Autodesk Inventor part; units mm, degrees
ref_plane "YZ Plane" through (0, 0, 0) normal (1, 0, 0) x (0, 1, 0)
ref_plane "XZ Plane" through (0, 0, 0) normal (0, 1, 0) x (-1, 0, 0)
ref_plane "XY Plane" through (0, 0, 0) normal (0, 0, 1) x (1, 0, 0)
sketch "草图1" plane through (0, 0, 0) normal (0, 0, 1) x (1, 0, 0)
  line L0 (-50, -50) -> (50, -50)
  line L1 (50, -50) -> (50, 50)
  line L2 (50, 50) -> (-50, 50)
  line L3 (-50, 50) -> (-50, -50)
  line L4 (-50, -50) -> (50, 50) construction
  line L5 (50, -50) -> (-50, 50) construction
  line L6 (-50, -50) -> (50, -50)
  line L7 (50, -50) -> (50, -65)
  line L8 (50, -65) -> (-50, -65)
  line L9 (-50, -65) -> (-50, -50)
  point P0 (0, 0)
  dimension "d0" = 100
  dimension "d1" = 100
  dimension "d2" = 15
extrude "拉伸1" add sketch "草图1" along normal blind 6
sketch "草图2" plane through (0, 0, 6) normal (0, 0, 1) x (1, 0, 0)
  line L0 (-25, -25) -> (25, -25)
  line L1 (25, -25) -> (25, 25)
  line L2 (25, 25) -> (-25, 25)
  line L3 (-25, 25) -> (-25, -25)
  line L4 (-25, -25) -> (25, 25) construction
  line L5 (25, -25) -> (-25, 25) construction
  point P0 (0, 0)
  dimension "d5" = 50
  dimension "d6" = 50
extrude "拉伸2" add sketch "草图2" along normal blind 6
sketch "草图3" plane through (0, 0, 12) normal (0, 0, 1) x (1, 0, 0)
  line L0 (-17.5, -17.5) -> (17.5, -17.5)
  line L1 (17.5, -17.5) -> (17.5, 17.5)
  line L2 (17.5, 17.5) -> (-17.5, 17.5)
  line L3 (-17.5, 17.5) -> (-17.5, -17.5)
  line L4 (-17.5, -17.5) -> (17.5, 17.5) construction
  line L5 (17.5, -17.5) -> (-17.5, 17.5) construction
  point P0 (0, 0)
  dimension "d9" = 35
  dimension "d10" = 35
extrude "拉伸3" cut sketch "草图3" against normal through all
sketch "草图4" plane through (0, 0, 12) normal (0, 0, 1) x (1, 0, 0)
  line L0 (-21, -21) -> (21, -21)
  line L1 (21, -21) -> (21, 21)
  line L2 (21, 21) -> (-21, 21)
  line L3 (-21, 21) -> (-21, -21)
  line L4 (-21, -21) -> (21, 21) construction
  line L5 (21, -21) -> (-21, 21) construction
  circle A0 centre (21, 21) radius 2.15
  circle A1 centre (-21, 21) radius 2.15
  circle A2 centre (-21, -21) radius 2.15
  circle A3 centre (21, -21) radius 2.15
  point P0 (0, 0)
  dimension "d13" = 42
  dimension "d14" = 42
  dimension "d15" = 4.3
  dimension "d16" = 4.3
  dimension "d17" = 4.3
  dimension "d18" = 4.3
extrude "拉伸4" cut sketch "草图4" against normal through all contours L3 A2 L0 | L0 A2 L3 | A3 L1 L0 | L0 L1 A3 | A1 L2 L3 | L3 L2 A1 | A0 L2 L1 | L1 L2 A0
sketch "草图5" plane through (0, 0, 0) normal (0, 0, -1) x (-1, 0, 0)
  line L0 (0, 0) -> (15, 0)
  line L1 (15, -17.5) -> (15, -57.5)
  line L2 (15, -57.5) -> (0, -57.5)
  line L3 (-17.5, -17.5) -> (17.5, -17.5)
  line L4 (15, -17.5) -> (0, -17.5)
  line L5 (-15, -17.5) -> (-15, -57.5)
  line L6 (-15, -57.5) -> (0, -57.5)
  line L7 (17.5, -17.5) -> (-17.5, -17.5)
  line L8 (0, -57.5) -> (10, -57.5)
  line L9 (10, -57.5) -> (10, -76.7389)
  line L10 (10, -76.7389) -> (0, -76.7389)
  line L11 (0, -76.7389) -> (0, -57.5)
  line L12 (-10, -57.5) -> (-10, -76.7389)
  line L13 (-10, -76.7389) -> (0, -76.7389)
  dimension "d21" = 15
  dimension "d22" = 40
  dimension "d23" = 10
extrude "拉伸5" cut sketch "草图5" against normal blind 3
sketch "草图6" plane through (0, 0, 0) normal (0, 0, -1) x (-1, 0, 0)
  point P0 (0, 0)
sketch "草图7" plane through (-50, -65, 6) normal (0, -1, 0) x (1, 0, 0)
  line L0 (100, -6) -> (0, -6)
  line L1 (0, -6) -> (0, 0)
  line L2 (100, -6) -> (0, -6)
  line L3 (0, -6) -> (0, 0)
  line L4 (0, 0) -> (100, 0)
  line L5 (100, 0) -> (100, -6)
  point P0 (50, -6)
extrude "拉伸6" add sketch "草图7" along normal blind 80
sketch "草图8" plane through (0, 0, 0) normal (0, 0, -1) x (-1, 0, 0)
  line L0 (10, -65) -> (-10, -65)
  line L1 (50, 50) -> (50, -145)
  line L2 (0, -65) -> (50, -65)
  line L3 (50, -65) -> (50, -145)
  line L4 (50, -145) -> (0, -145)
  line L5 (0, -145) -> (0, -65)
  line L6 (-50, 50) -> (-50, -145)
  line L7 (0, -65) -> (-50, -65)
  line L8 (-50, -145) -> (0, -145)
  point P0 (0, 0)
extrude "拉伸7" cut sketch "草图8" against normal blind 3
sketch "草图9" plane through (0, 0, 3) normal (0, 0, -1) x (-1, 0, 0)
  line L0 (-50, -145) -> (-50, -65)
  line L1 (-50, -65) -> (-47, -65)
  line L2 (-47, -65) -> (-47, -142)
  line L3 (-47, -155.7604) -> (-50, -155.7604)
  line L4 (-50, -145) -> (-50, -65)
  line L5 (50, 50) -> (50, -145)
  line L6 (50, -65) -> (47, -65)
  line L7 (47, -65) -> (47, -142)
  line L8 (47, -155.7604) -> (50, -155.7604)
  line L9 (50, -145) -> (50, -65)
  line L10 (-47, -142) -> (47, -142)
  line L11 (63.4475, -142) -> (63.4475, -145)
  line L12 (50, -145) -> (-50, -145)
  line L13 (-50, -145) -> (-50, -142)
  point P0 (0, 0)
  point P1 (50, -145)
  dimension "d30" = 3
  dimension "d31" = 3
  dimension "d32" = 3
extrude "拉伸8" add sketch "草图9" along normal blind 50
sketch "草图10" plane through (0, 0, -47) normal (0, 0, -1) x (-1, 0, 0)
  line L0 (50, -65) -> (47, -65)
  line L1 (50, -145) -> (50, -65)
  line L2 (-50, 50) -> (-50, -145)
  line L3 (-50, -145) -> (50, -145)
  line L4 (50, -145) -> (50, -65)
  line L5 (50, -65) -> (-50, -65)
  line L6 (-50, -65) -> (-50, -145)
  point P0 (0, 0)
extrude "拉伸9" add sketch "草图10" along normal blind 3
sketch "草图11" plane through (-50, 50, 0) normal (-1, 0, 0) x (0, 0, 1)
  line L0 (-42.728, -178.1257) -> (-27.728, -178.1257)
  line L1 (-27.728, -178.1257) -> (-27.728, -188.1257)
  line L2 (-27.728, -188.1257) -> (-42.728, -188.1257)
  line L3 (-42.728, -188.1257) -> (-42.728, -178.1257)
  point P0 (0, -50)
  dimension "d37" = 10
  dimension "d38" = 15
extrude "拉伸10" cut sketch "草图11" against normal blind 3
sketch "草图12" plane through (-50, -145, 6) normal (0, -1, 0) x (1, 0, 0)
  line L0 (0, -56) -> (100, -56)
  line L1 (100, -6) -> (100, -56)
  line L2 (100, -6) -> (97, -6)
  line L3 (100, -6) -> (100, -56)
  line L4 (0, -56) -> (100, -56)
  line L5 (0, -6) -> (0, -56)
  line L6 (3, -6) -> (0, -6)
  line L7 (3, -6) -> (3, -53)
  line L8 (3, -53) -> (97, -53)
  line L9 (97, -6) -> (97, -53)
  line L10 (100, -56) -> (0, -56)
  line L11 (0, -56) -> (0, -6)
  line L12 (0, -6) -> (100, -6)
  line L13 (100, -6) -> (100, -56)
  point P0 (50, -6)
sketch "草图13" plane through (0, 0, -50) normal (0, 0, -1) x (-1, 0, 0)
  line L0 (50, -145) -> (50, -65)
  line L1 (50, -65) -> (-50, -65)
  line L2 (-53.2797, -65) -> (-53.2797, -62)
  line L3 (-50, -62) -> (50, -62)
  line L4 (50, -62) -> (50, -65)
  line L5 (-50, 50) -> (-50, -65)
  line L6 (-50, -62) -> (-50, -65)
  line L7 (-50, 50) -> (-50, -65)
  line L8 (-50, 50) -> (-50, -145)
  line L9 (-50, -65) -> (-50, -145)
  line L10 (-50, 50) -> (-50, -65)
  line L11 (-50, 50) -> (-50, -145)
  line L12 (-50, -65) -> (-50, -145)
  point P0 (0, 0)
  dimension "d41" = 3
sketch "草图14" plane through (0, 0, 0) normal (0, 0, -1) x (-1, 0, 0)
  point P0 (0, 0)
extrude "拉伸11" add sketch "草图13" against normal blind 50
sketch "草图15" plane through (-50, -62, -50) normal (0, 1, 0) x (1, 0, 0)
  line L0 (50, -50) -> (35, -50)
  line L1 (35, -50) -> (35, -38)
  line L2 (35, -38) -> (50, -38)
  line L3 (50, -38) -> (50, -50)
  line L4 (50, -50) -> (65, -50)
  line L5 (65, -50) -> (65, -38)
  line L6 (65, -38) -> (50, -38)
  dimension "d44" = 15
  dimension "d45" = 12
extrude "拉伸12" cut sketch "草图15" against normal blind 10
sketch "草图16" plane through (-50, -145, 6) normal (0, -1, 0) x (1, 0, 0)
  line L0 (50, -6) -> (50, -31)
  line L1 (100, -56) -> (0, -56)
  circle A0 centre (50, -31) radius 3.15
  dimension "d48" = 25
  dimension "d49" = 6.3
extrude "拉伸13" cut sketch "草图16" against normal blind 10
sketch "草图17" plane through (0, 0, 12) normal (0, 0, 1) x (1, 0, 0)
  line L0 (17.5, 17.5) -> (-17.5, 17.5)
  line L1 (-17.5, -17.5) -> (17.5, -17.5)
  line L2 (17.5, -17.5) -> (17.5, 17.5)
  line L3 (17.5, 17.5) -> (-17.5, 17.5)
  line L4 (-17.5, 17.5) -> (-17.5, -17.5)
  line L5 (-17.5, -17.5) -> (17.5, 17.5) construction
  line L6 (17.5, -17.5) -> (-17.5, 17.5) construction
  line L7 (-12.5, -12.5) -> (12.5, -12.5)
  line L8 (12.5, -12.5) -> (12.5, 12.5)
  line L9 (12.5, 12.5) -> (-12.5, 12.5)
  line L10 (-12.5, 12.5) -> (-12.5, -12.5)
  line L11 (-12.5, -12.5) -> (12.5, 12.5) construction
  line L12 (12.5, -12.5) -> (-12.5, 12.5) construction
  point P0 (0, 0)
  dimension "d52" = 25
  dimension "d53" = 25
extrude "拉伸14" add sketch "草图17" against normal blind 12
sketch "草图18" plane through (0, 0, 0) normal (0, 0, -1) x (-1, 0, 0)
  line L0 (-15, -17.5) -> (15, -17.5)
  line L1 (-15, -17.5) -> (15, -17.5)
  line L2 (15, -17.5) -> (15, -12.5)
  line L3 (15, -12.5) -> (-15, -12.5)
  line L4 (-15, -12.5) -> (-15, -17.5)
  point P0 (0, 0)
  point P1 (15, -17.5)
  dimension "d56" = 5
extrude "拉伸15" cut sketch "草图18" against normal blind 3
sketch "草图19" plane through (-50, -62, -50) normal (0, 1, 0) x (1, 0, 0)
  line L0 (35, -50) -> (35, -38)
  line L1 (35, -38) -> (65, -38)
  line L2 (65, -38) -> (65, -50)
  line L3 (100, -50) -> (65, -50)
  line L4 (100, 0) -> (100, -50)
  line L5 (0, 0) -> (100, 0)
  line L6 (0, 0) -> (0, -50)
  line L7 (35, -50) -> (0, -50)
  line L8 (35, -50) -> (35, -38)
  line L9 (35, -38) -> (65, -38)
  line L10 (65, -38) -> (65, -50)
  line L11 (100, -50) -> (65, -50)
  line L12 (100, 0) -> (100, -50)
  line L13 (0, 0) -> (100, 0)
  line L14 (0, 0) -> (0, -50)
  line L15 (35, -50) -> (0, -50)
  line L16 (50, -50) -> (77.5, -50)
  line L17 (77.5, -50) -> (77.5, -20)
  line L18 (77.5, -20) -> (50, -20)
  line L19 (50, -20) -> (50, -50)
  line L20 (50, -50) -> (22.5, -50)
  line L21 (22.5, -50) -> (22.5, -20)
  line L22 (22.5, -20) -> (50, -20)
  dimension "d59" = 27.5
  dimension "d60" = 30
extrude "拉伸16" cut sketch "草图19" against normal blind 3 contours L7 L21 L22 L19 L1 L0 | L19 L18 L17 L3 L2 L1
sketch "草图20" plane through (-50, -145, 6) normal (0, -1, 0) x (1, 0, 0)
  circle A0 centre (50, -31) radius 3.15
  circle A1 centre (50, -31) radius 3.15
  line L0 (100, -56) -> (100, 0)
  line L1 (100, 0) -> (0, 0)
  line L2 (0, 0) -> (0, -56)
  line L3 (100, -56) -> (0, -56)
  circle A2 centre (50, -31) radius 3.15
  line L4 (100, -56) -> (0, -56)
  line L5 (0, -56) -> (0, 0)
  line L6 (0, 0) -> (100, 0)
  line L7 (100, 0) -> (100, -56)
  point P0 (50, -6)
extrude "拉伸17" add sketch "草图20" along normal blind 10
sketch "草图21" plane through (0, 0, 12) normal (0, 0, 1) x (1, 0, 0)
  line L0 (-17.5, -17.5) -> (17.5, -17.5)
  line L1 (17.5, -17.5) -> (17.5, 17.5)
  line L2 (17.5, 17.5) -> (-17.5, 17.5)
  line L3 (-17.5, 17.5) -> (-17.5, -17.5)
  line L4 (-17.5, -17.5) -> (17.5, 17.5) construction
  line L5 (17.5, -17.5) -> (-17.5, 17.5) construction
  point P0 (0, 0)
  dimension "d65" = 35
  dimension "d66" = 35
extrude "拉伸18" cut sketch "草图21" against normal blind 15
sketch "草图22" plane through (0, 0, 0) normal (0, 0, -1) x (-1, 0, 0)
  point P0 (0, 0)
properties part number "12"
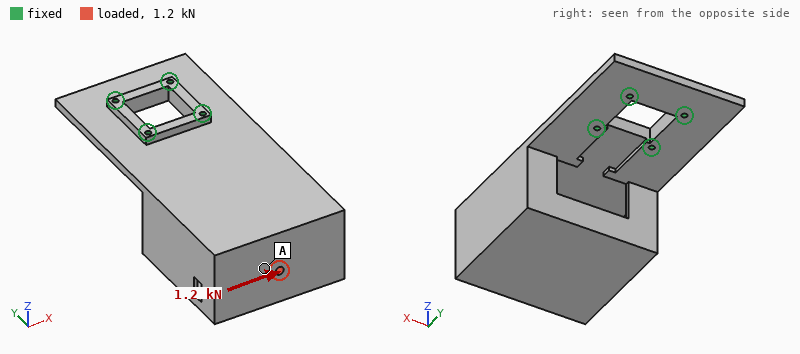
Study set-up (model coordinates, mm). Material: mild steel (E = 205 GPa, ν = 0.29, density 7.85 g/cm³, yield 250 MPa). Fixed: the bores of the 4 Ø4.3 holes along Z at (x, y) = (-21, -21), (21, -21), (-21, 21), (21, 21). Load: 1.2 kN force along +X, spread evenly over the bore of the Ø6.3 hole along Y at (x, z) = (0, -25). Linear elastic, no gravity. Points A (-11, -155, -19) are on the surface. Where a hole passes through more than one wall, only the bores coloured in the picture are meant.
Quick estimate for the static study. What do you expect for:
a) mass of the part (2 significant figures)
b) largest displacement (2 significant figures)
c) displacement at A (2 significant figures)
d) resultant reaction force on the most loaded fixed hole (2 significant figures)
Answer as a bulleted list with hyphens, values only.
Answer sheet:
- 1.7 kg
- 0.13 mm
- 0.058 mm
- 1.9 kN
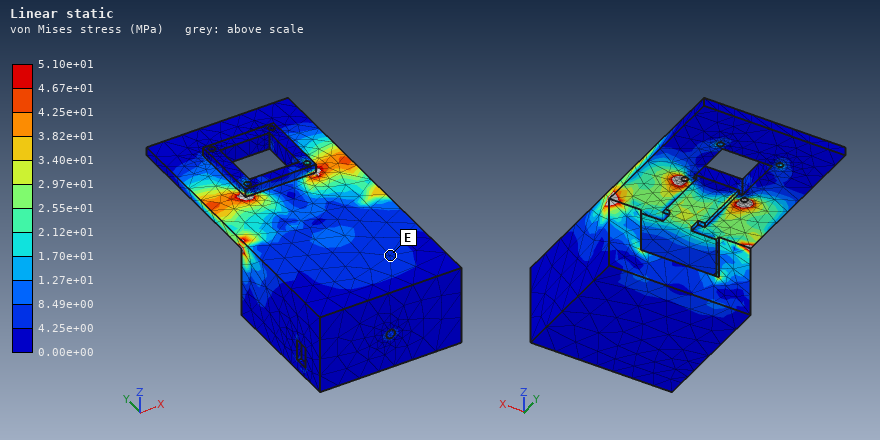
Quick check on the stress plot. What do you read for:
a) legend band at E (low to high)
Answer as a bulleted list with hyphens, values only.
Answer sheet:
- 4.25e+00 to 8.49e+00 MPa
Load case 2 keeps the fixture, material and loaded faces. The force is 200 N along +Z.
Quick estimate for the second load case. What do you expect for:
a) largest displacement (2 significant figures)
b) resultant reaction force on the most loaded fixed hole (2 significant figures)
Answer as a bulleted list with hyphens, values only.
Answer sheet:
- 0.50 mm
- 430 N
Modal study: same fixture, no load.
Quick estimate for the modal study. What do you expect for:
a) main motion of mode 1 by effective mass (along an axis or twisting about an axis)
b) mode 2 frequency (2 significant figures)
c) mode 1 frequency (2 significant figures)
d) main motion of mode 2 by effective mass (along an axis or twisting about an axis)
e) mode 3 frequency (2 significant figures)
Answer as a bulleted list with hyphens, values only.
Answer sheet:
- along Z
- 470 Hz
- 120 Hz
- along X
- 1100 Hz
